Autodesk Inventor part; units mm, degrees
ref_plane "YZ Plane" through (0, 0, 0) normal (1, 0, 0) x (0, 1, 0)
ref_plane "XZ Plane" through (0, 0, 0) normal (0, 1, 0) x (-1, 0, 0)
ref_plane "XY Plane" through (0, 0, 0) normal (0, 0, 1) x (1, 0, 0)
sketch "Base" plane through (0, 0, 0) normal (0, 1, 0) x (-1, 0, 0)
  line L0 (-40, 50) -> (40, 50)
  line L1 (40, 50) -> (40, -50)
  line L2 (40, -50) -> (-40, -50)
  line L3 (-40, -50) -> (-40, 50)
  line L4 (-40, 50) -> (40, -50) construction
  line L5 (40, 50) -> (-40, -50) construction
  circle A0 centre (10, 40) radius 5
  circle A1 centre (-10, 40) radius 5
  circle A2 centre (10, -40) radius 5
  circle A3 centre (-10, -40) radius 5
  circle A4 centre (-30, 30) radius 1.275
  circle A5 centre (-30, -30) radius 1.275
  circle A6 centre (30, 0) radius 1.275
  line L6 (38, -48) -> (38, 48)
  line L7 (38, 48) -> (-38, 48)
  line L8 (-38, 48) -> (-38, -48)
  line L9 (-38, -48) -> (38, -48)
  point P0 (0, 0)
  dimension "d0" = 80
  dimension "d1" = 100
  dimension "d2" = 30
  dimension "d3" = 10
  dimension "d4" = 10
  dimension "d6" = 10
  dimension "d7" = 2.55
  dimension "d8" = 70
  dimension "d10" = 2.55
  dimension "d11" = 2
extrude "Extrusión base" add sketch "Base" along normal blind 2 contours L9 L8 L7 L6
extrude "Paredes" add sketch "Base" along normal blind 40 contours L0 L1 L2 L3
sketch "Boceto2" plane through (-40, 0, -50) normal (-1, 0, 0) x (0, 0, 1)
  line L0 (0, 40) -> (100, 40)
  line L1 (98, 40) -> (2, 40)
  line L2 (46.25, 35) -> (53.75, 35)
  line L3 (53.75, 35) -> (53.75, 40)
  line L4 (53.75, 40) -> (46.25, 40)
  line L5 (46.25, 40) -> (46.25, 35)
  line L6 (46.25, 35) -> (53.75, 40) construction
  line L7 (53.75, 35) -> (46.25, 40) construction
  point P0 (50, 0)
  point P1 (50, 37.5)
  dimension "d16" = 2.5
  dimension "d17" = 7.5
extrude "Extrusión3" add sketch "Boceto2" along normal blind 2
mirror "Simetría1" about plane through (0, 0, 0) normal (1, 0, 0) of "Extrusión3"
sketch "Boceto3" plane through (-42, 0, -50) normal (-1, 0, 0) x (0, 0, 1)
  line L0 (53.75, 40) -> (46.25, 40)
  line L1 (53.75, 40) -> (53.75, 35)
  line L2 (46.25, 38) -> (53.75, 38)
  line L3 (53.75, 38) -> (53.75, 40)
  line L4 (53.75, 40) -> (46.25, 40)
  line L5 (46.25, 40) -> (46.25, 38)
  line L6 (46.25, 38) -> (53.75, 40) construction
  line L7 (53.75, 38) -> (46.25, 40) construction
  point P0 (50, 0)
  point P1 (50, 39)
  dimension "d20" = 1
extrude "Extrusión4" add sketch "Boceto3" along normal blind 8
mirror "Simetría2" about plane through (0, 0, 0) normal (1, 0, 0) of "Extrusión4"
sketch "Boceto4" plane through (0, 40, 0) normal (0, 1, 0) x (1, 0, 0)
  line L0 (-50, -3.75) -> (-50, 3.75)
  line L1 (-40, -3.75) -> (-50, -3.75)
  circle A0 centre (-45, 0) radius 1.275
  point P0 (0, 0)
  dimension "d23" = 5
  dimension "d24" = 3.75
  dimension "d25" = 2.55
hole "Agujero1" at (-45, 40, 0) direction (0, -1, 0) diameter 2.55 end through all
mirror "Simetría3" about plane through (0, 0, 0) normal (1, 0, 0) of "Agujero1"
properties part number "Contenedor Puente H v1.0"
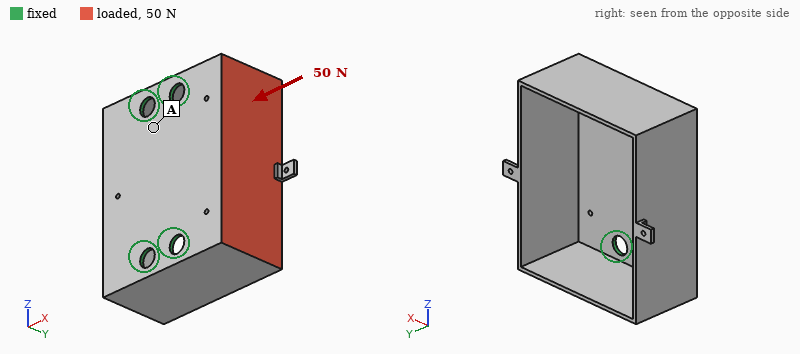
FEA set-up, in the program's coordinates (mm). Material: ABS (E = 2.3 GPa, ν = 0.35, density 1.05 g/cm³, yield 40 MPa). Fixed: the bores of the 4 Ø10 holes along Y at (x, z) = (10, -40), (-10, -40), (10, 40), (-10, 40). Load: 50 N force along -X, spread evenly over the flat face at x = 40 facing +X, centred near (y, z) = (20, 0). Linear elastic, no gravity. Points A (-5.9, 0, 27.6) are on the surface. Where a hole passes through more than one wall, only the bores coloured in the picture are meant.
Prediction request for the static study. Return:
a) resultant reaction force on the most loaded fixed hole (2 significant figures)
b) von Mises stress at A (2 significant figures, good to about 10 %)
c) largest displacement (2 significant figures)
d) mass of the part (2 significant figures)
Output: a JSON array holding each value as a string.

["23 N", "0.65 MPa", "1.6 mm", "45 g"]
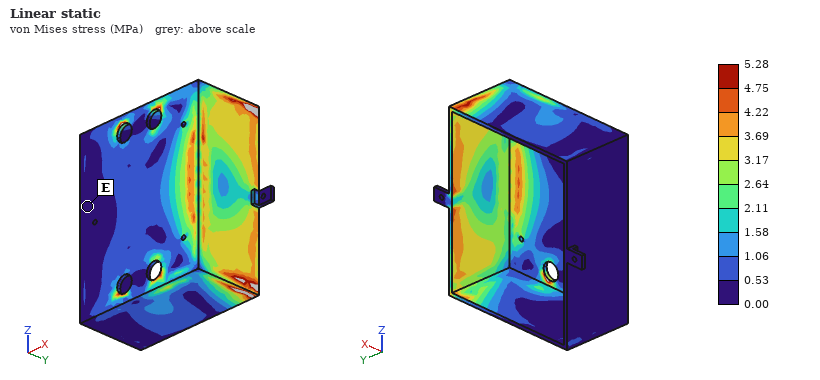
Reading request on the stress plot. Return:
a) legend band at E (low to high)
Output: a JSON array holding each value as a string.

["0.00 to 0.53 MPa"]
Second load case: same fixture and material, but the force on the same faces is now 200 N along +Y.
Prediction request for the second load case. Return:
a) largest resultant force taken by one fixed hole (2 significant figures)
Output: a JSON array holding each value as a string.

["210 N"]
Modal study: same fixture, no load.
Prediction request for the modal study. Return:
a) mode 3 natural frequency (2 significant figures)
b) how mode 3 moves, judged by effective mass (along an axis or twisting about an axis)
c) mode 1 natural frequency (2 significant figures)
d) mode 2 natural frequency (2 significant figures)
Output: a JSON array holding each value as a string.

["550 Hz", "along Z", "380 Hz", "380 Hz"]
